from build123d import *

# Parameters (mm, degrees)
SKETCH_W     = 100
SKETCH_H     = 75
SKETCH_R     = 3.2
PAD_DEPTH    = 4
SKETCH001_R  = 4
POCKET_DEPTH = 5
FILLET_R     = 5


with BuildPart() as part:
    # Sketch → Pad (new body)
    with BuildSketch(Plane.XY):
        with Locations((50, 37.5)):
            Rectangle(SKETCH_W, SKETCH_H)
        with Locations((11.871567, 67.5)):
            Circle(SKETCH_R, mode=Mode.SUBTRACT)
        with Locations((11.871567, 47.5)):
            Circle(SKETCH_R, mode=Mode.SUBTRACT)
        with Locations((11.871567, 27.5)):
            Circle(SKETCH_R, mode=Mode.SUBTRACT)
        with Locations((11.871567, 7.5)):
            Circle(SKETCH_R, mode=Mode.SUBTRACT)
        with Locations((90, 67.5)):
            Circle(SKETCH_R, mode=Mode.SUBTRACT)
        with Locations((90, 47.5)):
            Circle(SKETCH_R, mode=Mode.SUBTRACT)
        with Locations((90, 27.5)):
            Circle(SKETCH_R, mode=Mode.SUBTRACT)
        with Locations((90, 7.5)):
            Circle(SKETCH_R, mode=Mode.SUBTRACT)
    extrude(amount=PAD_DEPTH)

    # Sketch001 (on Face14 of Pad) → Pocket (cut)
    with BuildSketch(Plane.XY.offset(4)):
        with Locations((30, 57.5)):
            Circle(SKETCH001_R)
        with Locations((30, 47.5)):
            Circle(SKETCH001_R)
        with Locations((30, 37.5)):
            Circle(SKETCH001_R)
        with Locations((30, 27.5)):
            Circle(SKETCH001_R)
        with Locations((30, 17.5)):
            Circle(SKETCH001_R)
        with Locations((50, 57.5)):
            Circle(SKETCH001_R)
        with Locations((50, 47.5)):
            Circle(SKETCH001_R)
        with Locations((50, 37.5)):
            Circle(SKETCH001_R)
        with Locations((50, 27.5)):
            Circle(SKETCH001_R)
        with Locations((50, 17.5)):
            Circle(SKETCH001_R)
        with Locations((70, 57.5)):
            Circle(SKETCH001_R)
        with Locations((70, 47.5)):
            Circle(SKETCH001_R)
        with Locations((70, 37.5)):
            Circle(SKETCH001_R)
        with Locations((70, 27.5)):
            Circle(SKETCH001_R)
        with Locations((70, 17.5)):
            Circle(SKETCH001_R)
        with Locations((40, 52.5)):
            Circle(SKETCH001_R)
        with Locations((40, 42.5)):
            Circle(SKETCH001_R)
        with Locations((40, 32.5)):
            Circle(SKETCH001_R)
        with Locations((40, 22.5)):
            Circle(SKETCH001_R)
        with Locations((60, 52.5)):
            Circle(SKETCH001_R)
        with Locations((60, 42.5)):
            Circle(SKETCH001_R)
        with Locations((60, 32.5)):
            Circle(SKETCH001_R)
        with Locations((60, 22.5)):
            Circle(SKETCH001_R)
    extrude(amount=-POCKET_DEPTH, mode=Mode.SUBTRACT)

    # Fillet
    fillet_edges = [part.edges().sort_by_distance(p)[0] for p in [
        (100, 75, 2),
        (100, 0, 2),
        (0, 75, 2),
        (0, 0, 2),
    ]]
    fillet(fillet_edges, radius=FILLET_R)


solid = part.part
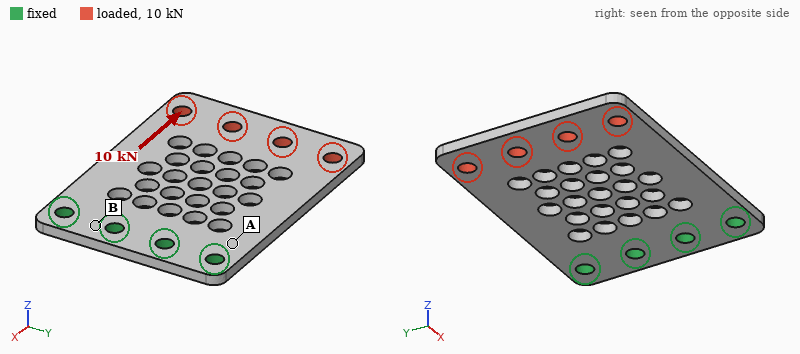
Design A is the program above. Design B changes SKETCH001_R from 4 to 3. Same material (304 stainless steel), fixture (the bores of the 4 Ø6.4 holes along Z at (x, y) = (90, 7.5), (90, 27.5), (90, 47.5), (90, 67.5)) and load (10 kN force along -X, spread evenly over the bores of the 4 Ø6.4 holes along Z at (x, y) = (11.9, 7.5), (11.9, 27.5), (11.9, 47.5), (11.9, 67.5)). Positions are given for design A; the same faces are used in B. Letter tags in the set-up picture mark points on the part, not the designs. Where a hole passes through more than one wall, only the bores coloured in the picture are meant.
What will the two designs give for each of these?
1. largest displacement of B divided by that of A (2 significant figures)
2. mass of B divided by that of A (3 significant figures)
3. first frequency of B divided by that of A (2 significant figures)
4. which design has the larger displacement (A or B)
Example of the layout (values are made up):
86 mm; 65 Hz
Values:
0.73; 1.08; 1.1; A
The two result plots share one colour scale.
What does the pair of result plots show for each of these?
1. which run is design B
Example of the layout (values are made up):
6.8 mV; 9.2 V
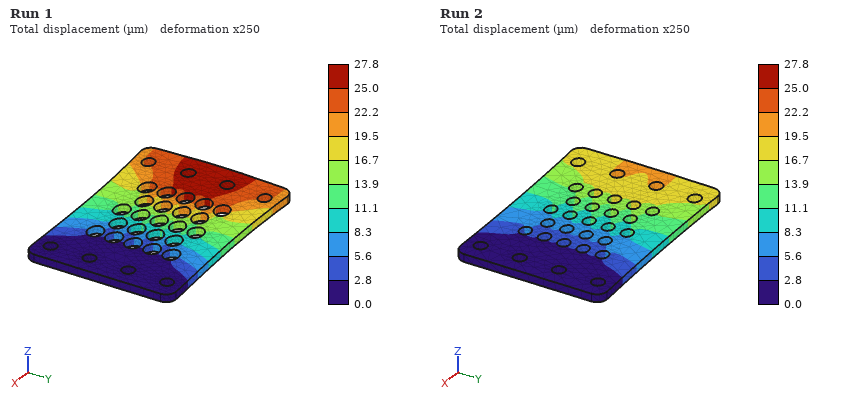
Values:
Run 2
